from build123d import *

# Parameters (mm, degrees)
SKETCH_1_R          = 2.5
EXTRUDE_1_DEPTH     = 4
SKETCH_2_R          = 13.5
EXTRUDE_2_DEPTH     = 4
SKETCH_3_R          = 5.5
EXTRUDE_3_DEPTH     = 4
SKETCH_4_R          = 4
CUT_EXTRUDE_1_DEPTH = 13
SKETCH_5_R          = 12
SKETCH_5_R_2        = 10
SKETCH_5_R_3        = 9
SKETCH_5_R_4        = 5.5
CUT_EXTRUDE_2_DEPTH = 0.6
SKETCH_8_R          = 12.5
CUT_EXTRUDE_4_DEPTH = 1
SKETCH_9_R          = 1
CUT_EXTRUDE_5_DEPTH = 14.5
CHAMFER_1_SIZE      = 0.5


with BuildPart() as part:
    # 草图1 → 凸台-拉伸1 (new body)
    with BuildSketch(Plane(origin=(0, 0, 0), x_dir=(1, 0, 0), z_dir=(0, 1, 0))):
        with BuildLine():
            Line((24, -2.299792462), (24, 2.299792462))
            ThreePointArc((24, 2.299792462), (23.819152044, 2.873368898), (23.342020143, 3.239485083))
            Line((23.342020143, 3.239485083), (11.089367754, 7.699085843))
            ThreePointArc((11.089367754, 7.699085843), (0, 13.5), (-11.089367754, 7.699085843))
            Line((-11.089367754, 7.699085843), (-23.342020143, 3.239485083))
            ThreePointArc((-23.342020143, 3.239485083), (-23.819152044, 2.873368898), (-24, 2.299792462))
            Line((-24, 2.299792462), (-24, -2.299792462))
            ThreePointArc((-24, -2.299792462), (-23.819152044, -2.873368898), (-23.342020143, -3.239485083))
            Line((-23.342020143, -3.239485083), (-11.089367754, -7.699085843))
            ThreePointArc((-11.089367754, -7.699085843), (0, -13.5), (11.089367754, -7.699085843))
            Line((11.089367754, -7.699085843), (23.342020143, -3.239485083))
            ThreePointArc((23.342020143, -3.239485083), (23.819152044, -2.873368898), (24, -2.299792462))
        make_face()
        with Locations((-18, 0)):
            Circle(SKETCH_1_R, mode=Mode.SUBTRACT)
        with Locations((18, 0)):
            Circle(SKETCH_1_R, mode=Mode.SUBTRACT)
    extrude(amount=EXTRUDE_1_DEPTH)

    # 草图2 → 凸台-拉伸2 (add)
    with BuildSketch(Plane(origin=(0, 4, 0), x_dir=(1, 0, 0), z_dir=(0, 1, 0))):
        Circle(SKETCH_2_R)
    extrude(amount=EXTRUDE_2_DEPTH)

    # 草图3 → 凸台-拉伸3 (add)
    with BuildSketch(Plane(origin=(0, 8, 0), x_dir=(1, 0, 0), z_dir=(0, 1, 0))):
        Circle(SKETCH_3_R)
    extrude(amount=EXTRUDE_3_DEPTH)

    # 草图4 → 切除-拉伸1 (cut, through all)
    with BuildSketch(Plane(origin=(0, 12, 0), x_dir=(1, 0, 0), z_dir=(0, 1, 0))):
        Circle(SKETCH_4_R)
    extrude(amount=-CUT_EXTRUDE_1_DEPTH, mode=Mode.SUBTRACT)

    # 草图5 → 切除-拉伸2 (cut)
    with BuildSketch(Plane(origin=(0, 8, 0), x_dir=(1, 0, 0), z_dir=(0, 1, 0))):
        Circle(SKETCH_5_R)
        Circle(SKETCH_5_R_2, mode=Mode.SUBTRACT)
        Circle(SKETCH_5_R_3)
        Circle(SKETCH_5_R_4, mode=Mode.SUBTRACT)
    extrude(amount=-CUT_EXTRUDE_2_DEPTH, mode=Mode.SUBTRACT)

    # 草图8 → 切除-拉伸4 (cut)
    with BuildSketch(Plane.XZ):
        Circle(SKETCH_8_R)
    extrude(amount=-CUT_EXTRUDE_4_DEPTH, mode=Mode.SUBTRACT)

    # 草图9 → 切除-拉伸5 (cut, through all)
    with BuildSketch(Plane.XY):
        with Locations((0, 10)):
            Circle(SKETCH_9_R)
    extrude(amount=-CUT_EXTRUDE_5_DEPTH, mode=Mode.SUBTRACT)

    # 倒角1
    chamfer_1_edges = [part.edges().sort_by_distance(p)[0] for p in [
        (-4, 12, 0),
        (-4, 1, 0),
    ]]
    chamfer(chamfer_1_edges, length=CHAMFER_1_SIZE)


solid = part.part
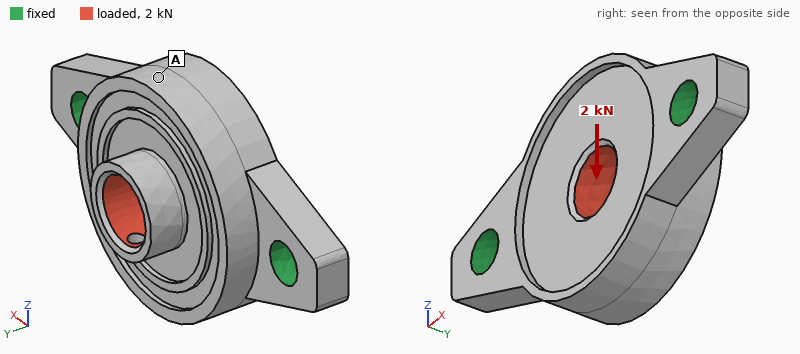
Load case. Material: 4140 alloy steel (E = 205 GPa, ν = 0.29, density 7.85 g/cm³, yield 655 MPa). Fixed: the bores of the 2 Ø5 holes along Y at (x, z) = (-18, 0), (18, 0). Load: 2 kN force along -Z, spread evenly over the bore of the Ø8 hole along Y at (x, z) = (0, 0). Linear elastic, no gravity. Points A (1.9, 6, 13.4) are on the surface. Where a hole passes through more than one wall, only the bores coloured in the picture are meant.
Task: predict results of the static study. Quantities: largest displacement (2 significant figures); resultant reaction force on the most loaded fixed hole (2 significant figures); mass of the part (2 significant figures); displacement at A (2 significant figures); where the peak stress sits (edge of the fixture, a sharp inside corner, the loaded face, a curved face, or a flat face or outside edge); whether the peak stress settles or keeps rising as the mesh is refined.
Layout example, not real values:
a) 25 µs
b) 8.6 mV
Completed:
a) 18 µm
b) 1.0 kN
c) 35 g
d) 17 µm
e) edge of the fixture
f) keeps rising
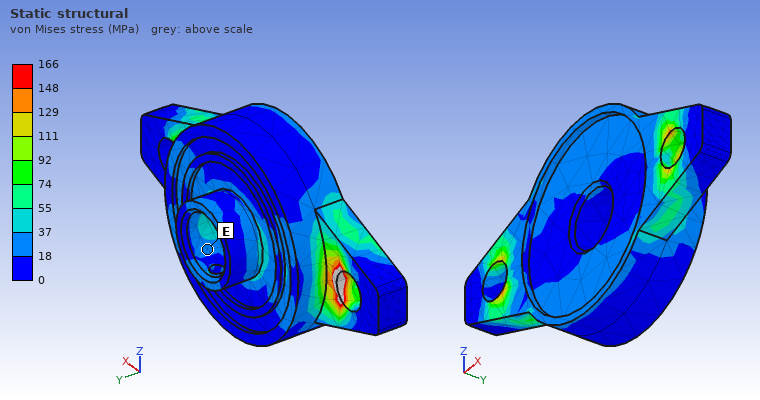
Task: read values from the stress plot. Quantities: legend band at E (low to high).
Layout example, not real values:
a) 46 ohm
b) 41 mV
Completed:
a) 18 to 37 MPa
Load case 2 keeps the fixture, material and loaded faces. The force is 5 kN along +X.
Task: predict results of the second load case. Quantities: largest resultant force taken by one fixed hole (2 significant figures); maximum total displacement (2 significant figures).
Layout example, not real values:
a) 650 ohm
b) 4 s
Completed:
a) 2.6 kN
b) 8.4 µm
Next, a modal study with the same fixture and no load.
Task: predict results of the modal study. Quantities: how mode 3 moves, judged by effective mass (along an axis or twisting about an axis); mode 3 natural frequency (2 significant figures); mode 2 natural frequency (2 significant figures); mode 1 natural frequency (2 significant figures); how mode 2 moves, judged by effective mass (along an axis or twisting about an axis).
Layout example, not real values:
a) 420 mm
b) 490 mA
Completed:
a) along Z
b) 28 kHz
c) 16 kHz
d) 10 kHz
e) along Y
